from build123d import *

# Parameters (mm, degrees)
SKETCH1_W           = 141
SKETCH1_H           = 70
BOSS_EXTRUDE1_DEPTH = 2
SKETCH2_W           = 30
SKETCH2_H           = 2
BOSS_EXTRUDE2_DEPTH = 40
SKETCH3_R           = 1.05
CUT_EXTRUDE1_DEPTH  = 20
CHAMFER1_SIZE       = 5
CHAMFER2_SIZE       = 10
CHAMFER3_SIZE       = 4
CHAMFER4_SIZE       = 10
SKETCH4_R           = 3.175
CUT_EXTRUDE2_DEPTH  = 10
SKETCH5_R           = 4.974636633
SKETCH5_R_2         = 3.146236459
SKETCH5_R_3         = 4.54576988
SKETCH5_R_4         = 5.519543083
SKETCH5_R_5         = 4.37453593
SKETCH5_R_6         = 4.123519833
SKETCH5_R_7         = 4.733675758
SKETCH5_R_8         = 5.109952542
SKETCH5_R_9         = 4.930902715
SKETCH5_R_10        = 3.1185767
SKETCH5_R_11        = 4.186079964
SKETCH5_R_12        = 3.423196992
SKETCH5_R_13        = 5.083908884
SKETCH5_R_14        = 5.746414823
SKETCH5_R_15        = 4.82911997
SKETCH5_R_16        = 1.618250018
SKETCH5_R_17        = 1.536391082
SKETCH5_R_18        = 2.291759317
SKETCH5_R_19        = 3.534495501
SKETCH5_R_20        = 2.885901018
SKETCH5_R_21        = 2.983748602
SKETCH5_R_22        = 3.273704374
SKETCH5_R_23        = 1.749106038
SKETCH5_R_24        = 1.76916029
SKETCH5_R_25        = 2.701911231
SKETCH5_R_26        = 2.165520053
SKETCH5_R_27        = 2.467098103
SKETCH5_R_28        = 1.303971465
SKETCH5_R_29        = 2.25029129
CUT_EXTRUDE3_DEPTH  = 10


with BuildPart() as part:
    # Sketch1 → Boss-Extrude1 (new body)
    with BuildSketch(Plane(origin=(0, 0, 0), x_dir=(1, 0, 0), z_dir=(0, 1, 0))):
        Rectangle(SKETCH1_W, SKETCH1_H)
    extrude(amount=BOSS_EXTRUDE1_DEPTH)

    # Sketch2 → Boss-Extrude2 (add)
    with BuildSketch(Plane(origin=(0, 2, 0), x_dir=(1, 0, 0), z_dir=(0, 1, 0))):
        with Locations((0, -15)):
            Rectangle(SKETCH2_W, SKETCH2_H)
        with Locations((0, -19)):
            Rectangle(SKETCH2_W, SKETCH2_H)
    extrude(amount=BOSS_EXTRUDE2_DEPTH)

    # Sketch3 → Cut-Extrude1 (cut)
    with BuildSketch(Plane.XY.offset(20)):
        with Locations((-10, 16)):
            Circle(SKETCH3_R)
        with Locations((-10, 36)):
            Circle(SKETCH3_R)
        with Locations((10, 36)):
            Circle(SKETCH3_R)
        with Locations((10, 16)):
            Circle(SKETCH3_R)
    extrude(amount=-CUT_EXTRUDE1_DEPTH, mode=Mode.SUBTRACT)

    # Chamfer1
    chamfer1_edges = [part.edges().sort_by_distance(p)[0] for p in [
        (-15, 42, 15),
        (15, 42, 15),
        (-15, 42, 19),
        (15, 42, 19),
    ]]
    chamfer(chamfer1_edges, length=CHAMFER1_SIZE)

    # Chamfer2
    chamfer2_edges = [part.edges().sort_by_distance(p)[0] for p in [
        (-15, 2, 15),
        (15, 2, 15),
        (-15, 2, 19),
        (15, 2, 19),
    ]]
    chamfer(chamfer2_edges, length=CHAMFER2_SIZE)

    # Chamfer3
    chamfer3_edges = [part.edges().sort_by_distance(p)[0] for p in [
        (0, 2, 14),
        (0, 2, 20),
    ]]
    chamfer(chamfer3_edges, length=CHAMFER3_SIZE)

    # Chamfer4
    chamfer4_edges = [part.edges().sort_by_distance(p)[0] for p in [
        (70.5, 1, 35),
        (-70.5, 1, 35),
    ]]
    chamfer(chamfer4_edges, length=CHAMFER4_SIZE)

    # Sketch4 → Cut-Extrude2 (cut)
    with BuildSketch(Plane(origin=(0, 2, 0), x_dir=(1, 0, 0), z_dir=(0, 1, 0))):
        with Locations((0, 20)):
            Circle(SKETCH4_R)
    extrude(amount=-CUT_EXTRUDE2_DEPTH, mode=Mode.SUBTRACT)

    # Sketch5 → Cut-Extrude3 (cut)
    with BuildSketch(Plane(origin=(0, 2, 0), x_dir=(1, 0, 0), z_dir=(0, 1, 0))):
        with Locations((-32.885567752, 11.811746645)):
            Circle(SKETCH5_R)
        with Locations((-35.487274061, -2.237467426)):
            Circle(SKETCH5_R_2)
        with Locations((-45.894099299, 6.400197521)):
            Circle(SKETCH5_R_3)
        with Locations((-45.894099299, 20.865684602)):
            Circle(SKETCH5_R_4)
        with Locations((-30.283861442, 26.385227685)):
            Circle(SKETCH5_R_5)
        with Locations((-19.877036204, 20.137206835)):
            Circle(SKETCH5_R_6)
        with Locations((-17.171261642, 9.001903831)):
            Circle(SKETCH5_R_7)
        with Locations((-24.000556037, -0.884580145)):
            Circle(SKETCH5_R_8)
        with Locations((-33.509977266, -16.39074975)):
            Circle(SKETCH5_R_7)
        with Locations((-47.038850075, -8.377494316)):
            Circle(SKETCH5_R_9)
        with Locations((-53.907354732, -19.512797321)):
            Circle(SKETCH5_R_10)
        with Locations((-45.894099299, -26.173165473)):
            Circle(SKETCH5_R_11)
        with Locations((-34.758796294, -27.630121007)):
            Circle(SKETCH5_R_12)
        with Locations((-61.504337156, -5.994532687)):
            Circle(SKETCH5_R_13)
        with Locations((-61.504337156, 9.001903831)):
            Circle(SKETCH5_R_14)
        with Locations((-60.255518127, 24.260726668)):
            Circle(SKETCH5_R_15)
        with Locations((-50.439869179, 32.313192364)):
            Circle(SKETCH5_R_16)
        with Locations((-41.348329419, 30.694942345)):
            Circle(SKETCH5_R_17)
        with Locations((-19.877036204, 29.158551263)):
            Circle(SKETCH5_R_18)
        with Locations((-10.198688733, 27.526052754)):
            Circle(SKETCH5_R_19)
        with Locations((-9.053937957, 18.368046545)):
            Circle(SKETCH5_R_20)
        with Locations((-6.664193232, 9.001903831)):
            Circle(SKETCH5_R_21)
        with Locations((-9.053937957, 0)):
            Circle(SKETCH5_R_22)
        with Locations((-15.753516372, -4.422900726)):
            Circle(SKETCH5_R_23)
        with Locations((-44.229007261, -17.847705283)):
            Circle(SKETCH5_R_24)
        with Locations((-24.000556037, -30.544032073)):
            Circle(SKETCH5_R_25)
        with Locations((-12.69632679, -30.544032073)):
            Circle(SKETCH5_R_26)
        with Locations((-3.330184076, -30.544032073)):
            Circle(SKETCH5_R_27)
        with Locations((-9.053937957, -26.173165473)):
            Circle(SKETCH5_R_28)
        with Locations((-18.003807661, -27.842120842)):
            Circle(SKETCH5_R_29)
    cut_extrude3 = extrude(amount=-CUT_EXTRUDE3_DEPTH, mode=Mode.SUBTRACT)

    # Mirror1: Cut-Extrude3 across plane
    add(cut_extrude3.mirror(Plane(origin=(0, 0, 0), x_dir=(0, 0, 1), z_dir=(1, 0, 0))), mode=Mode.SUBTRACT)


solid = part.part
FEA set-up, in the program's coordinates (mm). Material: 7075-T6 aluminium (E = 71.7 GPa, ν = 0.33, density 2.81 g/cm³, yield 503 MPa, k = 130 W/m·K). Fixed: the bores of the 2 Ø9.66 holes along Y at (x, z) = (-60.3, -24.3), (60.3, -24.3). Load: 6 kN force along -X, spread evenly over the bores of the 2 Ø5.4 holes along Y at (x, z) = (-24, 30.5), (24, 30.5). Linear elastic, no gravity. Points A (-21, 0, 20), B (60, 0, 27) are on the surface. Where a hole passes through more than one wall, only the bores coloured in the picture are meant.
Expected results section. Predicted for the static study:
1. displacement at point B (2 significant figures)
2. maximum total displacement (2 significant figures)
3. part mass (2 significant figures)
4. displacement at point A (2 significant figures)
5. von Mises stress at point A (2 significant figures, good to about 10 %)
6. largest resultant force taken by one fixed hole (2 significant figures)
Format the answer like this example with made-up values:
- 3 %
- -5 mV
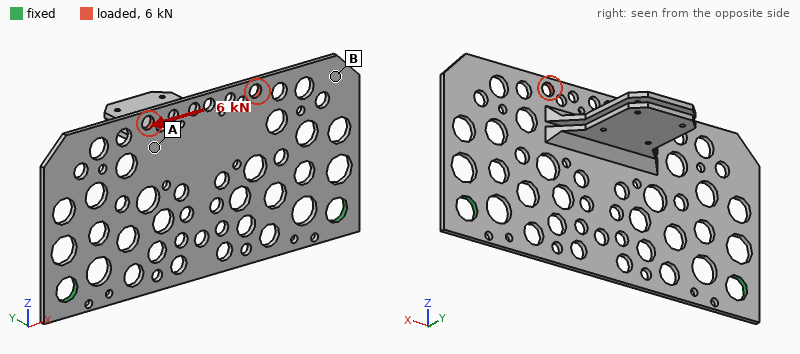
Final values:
- 0.17 mm
- 0.20 mm
- 56 g
- 0.14 mm
- 69 MPa
- 4.0 kN
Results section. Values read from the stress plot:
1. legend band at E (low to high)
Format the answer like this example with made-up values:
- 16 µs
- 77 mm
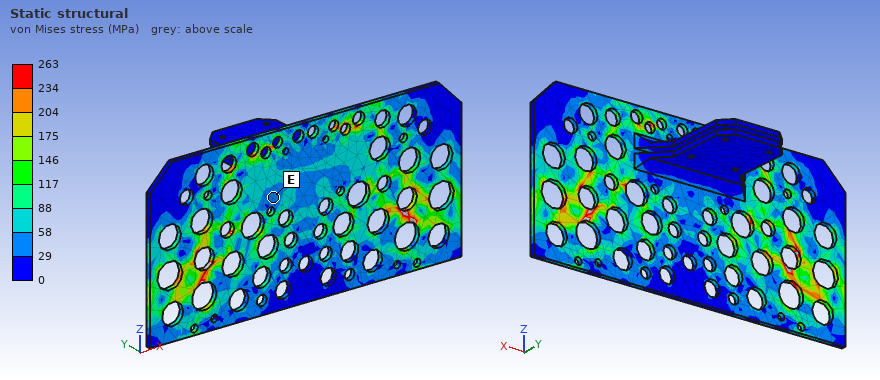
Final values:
- 29 to 58 MPa
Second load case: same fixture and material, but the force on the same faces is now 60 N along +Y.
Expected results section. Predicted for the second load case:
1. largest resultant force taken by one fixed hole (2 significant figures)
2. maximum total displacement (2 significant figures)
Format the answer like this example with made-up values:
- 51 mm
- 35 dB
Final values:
- 30 N
- 1.6 mm
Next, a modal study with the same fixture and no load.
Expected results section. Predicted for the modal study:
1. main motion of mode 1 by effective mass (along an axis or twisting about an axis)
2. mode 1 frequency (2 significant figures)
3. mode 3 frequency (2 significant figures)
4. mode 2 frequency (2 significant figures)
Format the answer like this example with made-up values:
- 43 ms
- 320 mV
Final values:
- along Y
- 220 Hz
- 630 Hz
- 610 Hz
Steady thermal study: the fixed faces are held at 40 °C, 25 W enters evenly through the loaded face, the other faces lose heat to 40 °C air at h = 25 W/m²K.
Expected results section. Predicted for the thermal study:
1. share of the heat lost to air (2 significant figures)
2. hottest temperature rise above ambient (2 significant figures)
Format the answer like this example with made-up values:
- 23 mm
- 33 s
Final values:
- 65 %
- 75 K
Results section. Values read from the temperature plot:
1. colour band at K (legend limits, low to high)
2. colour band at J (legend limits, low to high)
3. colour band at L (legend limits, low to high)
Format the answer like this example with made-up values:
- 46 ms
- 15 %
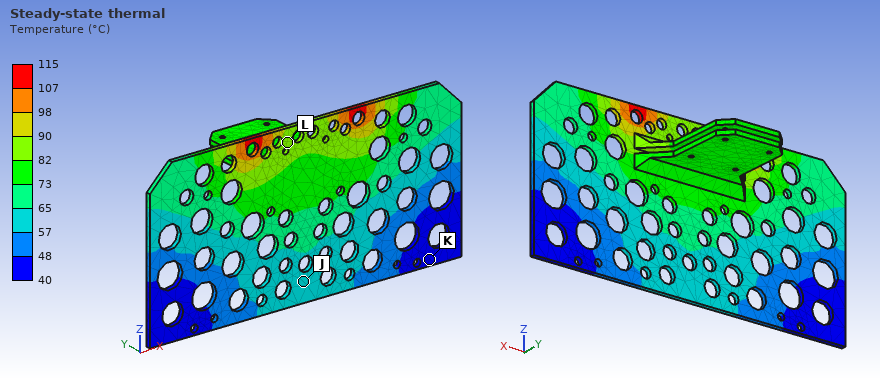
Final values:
- 40 to 48 °C
- 57 to 65 °C
- 82 to 90 °C
